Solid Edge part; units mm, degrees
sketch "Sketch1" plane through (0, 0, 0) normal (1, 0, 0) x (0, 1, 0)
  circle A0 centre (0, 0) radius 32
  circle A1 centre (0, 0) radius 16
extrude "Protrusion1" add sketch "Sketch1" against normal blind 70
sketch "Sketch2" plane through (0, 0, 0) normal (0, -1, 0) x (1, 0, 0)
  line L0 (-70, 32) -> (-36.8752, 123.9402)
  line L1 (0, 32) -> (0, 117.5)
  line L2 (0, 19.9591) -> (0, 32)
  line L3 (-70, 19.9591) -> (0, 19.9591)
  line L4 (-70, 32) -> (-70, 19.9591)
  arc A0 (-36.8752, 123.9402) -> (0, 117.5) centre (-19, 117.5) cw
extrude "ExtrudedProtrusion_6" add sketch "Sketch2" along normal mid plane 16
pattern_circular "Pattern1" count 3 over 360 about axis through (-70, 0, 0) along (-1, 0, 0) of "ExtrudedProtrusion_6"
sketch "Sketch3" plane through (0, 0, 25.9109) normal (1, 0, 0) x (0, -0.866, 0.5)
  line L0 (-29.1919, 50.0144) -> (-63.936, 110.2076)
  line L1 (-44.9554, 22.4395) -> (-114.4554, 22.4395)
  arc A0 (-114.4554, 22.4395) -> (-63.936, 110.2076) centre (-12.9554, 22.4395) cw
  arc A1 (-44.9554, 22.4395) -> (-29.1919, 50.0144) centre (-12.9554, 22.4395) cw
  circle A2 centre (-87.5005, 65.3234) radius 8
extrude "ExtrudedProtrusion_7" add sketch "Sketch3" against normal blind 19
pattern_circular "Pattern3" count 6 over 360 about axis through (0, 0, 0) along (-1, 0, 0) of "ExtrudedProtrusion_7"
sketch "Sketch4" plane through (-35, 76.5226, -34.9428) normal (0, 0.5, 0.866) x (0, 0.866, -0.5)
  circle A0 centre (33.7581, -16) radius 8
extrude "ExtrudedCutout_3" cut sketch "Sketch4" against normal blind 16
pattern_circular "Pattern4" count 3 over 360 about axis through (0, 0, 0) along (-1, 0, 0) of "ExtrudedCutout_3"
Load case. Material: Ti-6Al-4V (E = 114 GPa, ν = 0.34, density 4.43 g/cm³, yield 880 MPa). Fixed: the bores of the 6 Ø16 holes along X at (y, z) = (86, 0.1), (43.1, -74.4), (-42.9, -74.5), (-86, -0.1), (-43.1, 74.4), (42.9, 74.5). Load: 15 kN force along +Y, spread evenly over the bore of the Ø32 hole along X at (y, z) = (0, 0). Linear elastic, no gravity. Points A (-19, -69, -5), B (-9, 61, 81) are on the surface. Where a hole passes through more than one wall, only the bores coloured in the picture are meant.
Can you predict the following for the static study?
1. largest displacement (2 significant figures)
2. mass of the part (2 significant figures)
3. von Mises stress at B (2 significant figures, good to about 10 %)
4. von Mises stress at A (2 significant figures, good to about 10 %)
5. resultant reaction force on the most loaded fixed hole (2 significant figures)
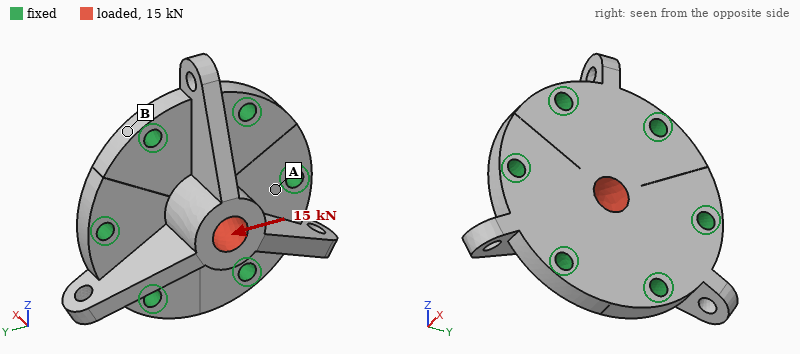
11 µm
3.9 kg
2.2 MPa
7.0 MPa
4.4 kN
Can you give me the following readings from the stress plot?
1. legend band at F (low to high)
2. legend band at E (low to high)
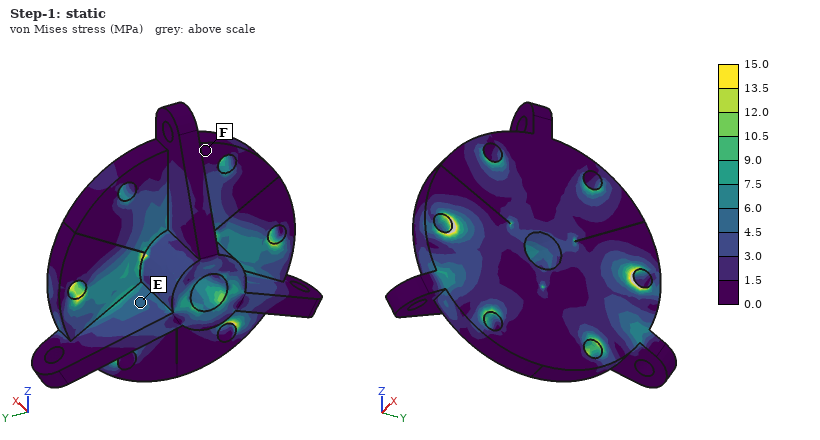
0.0 to 1.5 MPa
4.5 to 6.0 MPa
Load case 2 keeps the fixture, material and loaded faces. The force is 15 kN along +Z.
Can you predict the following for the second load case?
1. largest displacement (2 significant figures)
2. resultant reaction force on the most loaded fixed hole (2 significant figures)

12 µm
3.9 kN
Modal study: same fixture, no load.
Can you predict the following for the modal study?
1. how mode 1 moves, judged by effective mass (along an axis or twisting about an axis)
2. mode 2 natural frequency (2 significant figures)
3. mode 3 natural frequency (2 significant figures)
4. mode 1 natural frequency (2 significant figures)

along X
5400 Hz
5400 Hz
5000 Hz
